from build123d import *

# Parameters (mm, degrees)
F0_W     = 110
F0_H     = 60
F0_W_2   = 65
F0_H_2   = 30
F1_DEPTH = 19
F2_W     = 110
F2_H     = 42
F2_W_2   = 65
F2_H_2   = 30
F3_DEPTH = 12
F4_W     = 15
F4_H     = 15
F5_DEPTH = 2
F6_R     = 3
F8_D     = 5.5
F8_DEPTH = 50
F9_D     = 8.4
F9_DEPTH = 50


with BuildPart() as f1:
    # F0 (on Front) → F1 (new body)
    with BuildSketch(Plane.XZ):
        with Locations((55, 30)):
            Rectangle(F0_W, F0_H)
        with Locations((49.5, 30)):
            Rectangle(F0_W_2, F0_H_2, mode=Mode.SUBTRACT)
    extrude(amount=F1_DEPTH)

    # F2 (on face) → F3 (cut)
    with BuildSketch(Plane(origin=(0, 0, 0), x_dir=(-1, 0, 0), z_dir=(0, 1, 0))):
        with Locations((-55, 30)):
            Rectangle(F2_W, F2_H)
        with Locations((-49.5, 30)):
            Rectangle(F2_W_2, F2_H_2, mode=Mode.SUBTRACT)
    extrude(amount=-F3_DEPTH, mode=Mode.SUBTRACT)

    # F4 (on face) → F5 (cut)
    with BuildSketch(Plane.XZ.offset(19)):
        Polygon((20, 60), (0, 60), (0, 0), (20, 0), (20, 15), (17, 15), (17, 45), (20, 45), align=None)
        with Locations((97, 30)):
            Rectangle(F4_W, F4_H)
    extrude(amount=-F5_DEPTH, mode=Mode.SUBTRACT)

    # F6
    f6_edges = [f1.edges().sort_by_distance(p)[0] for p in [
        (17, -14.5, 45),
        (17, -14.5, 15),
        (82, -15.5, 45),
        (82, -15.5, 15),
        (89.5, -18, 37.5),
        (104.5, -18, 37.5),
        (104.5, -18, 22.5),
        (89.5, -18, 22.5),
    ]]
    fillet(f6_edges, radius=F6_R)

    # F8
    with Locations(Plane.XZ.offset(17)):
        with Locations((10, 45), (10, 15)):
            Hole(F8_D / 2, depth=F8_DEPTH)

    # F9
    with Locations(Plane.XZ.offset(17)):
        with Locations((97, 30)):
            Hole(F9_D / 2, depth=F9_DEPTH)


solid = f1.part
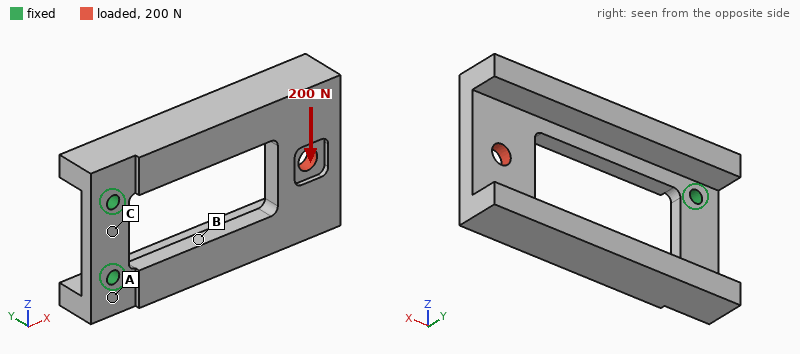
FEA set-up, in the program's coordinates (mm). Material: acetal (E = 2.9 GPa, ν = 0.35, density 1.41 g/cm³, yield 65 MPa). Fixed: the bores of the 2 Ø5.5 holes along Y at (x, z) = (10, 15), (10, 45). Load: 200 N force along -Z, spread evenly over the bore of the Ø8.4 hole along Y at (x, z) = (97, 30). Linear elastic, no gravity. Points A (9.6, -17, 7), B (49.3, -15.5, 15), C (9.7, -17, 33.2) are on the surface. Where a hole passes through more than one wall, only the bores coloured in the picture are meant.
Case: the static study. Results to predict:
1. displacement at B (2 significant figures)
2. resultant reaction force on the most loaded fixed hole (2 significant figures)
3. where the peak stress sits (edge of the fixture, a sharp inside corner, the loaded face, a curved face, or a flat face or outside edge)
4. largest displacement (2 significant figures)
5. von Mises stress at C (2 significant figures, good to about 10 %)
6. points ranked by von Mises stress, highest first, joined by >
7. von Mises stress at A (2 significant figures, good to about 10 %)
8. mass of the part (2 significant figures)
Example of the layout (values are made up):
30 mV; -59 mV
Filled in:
0.57 mm; 400 N; edge of the fixture; 1.3 mm; 5.5 MPa; A > C > B; 9.6 MPa; 75 g
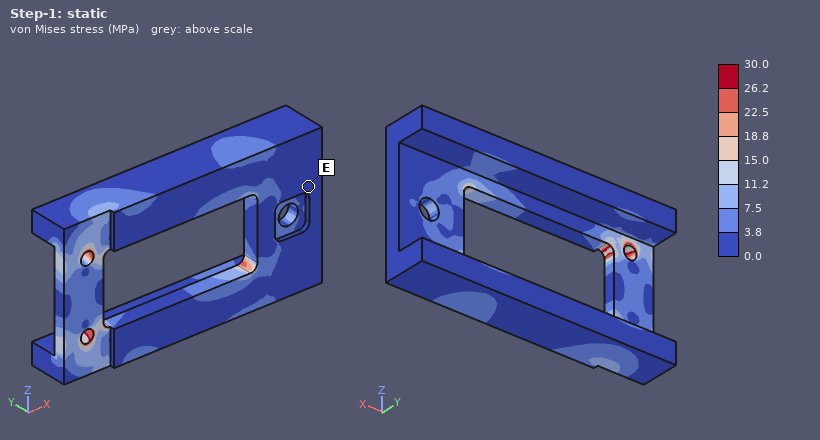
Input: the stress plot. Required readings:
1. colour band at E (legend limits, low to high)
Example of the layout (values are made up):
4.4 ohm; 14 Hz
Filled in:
0.0 to 3.8 MPa
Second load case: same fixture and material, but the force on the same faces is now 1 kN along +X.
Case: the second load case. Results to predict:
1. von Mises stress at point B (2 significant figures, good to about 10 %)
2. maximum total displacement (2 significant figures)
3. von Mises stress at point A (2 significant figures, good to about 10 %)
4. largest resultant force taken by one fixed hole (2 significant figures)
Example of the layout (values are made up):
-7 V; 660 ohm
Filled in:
6.8 MPa; 0.47 mm; 5.6 MPa; 500 N
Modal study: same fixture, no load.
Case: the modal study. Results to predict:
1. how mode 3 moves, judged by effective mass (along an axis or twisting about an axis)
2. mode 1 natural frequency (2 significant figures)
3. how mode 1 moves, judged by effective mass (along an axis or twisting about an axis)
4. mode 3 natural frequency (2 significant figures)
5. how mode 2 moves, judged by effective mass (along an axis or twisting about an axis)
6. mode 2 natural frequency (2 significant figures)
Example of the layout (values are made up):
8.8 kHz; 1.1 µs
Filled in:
along Z; 160 Hz; along Y; 380 Hz; along Z; 310 Hz
